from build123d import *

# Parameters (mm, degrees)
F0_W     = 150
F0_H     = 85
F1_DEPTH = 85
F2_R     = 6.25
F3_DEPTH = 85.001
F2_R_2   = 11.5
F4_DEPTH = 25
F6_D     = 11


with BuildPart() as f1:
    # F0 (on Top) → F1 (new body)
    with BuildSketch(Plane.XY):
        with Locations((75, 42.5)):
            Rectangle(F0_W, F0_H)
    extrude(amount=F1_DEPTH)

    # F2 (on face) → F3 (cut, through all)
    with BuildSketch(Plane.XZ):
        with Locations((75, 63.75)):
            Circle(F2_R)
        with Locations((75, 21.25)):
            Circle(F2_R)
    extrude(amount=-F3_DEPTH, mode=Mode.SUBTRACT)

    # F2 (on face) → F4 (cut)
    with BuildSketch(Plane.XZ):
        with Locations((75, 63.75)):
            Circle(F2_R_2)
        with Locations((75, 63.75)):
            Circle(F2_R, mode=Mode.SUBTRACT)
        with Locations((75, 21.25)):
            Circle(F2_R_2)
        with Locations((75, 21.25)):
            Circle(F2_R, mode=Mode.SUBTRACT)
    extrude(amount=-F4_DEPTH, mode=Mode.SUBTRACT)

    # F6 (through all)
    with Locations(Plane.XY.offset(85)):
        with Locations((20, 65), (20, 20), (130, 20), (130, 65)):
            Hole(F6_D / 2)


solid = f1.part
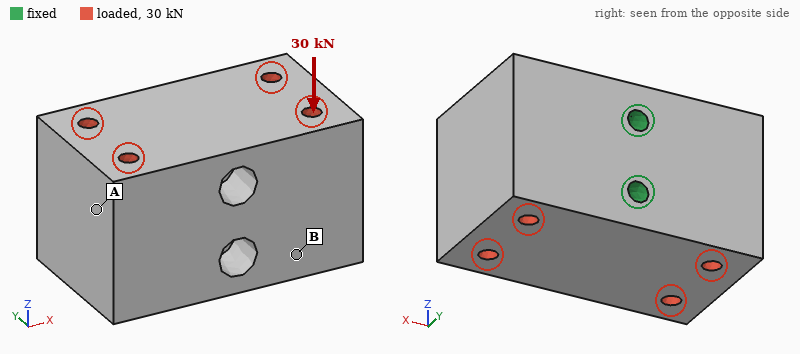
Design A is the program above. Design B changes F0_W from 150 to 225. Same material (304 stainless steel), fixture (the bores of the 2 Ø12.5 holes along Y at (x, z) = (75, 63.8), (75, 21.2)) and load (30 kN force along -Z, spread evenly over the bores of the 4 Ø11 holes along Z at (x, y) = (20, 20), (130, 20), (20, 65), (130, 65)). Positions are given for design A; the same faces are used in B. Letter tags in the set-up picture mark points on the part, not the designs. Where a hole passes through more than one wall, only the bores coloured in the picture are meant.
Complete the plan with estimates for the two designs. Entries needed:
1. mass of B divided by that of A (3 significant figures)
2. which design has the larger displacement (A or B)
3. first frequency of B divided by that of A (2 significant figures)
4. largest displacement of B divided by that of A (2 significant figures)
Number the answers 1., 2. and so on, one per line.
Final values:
1. 1.53
2. B
3. 0.55
4. 1.2
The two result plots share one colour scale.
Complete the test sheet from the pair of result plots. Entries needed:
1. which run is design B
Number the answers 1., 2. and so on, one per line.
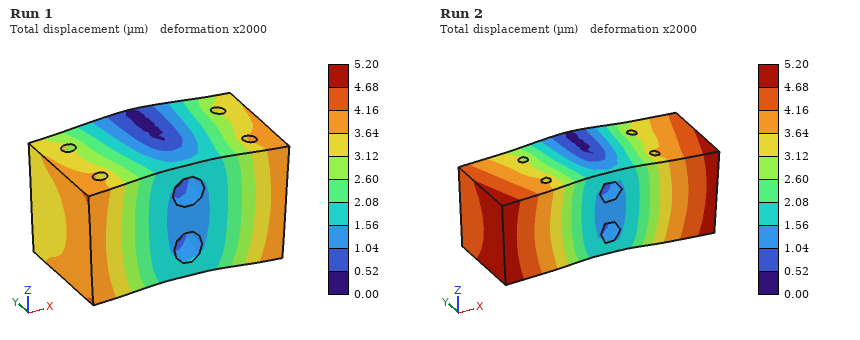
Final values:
1. Run 2
